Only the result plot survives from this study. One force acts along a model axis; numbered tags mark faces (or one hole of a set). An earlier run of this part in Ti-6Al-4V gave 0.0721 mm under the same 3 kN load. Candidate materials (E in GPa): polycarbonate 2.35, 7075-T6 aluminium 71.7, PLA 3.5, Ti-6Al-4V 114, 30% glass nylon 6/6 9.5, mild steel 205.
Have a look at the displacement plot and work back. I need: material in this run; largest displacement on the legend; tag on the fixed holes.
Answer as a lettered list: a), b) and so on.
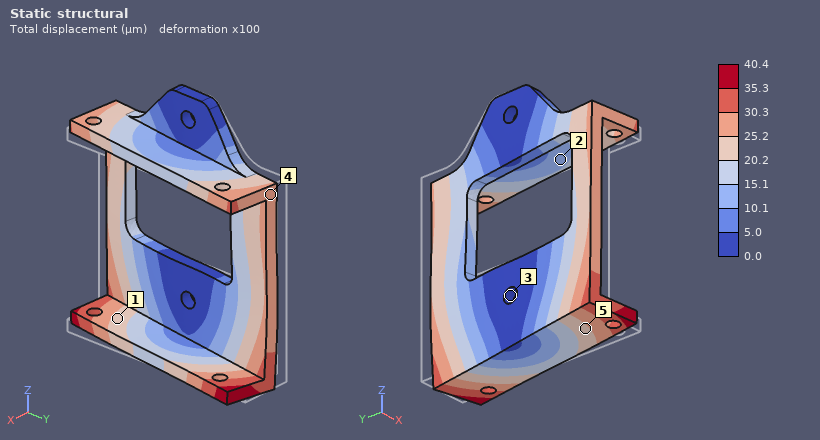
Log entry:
a) mild steel
b) 40.4 µm
c) 3
